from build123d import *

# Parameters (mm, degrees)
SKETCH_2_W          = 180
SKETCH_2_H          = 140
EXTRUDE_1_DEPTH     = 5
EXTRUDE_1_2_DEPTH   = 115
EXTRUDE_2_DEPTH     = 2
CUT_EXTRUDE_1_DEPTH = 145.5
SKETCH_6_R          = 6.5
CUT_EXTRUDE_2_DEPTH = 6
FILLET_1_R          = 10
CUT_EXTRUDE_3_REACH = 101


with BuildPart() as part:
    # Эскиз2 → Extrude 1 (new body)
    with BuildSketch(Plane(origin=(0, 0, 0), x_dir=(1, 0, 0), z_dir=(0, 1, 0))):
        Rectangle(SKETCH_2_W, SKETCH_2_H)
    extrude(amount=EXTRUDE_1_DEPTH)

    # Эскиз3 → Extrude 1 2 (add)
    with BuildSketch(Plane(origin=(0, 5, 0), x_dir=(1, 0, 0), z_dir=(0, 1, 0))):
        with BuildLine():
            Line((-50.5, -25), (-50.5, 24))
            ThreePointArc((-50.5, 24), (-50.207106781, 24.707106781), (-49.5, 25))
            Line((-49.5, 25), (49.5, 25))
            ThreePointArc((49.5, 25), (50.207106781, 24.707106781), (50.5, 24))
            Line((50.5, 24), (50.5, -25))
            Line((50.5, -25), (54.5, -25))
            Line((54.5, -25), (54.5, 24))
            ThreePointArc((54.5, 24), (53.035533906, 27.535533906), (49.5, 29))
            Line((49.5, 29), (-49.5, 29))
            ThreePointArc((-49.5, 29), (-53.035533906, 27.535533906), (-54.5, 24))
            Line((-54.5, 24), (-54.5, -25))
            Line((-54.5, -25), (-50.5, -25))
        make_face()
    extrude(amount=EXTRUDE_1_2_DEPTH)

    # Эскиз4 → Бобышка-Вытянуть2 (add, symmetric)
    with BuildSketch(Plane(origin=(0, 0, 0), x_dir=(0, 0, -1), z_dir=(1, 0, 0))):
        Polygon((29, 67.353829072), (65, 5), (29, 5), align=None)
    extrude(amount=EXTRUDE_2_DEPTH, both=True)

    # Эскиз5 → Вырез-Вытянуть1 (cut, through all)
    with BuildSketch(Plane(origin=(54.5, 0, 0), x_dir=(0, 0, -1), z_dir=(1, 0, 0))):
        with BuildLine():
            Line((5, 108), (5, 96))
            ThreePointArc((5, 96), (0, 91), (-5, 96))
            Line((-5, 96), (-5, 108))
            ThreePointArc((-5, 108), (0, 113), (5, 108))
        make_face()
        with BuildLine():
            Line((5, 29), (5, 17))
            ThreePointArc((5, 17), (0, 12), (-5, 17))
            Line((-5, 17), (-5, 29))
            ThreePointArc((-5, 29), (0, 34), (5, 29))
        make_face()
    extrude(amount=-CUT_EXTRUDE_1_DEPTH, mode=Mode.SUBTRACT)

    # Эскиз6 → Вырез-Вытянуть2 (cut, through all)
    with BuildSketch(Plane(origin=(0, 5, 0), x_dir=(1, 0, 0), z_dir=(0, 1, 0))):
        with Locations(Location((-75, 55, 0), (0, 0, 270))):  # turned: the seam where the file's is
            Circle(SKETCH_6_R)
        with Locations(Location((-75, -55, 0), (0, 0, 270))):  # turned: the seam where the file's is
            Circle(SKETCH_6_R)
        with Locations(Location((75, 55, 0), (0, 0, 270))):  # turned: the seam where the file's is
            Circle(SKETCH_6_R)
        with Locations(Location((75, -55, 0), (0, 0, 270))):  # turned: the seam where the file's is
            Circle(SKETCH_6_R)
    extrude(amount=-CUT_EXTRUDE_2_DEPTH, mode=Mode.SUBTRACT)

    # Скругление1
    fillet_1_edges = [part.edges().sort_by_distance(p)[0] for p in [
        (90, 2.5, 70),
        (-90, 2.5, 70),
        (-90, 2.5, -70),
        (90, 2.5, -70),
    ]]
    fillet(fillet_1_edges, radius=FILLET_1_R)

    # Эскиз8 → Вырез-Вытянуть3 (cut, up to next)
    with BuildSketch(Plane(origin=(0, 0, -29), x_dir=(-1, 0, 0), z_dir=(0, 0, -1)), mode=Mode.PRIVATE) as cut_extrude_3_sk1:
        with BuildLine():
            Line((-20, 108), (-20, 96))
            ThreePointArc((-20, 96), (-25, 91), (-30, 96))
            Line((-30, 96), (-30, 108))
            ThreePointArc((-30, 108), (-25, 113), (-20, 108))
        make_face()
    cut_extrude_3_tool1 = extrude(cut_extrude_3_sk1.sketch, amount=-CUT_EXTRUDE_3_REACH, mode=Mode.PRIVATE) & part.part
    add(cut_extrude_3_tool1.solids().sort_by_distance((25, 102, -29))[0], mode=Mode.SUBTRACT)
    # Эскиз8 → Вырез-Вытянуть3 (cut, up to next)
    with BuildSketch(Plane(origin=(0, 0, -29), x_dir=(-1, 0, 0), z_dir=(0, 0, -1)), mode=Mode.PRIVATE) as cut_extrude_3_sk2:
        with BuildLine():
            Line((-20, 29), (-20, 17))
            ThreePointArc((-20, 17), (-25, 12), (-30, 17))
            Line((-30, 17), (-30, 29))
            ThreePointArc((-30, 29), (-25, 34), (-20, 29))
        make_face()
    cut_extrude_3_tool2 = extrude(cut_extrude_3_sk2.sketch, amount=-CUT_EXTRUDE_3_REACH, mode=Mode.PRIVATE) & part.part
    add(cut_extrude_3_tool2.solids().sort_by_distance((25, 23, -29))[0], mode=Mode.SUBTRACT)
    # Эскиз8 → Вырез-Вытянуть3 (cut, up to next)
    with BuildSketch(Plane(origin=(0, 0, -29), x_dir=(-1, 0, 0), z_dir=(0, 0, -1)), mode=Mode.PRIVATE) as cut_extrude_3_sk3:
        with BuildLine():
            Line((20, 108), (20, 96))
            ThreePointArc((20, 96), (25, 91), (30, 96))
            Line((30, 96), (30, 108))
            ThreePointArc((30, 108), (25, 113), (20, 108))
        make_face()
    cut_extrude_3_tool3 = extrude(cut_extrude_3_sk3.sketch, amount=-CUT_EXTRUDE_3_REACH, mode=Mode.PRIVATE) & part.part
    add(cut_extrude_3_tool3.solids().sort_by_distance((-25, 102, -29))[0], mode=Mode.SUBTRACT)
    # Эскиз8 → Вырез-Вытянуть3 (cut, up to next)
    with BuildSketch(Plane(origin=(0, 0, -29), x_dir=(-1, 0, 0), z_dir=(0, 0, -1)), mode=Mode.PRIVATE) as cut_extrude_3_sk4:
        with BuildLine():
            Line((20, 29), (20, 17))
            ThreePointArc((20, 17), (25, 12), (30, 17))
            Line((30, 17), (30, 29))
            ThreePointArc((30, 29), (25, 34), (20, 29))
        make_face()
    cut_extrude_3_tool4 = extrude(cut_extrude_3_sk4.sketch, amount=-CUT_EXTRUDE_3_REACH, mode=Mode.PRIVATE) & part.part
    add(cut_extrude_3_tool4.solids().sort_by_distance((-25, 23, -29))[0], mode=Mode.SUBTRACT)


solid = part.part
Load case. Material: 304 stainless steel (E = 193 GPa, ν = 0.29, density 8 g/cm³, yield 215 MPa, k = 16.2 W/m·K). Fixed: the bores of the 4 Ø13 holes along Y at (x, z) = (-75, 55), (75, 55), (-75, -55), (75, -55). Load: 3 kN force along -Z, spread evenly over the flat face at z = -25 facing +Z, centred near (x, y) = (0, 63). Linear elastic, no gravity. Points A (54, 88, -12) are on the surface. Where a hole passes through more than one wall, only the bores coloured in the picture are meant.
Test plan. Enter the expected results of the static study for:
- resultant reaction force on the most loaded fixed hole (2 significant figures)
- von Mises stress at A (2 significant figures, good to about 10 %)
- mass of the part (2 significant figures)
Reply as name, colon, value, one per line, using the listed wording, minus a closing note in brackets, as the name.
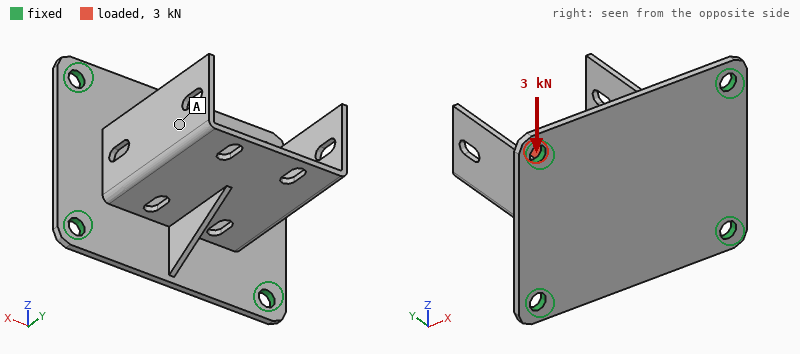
resultant reaction force on the most loaded fixed hole: 1.3 kN
von Mises stress at A: 30 MPa
mass of the part: 1.7 kg
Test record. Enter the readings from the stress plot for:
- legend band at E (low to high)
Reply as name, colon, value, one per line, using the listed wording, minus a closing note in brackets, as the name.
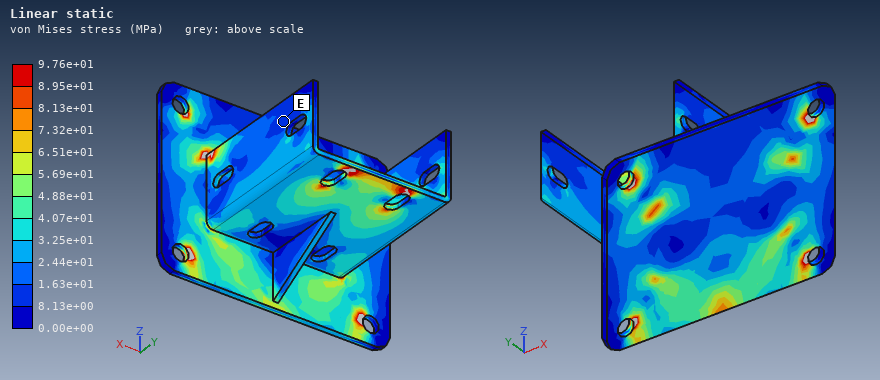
legend band at E: 8.13e+00 to 1.63e+01 MPa
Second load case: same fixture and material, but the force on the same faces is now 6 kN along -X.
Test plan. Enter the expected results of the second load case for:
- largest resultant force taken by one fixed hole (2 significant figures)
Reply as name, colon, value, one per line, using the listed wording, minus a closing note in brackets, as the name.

largest resultant force taken by one fixed hole: 3.2 kN
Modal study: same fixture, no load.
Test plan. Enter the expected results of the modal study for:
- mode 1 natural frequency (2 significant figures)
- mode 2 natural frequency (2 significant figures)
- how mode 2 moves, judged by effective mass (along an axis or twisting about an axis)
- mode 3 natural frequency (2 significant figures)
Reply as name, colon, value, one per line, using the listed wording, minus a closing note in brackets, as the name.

mode 1 natural frequency: 730 Hz
mode 2 natural frequency: 760 Hz
how mode 2 moves, judged by effective mass: along X
mode 3 natural frequency: 920 Hz
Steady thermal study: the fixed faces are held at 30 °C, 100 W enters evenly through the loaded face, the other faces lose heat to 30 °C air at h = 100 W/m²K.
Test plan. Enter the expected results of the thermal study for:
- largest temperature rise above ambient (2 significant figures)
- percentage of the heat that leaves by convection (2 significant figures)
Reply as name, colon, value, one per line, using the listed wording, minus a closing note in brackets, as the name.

largest temperature rise above ambient: 72 K
percentage of the heat that leaves by convection: 99 %
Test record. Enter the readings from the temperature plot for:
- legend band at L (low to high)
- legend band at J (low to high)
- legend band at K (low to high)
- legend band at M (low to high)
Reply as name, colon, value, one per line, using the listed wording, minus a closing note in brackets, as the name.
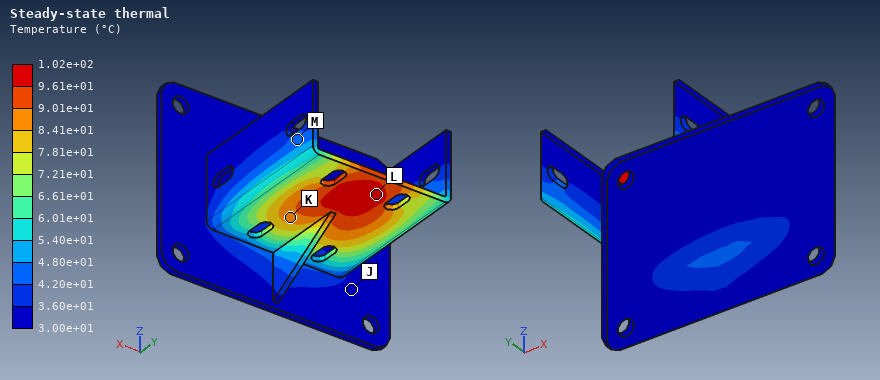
legend band at L: 9.61e+01 to 1.02e+02 °C
legend band at J: 3.00e+01 to 3.60e+01 °C
legend band at K: 8.41e+01 to 9.01e+01 °C
legend band at M: 4.20e+01 to 4.80e+01 °C
